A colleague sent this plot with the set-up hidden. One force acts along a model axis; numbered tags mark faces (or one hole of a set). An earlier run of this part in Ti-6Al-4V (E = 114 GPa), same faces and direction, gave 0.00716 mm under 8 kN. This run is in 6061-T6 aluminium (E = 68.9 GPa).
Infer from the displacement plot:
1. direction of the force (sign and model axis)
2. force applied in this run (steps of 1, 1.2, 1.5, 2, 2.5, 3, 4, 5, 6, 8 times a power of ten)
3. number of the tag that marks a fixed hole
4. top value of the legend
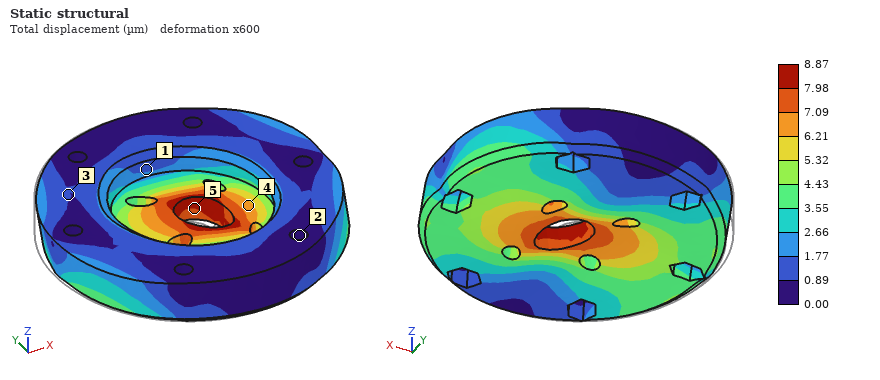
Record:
+X
6 kN
2
8.87 µm
